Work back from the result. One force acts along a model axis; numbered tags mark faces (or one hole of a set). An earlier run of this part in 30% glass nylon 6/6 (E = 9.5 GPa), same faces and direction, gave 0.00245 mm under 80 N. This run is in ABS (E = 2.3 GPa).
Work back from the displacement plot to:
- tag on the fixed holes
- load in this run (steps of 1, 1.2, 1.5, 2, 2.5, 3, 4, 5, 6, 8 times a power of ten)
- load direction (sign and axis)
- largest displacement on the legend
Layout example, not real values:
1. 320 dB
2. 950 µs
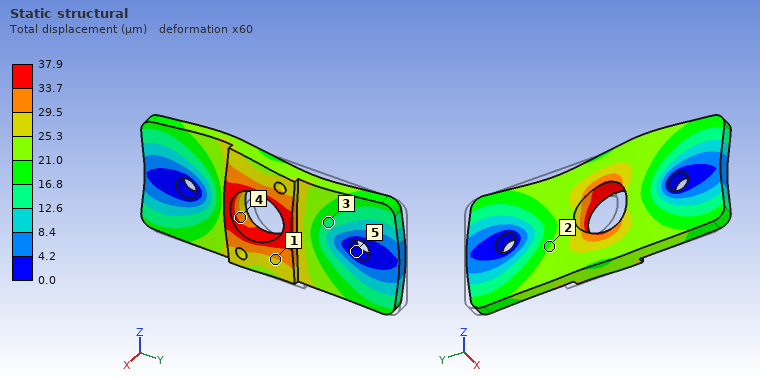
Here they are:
1. 5
2. 300 N
3. -Y
4. 37.9 µm
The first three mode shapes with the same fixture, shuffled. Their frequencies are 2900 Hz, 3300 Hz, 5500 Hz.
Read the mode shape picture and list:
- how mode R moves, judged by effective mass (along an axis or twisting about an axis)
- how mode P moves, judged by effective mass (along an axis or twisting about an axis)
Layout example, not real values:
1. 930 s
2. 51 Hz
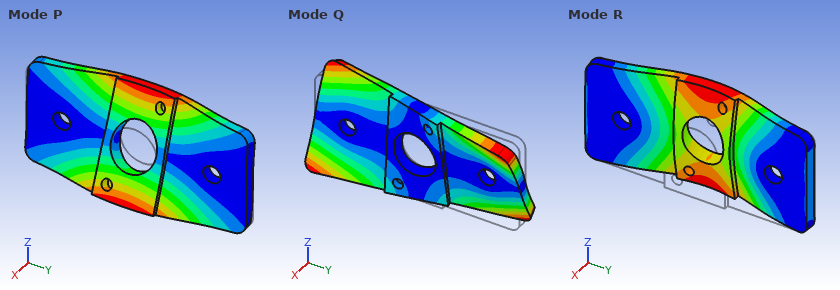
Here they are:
1. along X
2. twisting about Y
